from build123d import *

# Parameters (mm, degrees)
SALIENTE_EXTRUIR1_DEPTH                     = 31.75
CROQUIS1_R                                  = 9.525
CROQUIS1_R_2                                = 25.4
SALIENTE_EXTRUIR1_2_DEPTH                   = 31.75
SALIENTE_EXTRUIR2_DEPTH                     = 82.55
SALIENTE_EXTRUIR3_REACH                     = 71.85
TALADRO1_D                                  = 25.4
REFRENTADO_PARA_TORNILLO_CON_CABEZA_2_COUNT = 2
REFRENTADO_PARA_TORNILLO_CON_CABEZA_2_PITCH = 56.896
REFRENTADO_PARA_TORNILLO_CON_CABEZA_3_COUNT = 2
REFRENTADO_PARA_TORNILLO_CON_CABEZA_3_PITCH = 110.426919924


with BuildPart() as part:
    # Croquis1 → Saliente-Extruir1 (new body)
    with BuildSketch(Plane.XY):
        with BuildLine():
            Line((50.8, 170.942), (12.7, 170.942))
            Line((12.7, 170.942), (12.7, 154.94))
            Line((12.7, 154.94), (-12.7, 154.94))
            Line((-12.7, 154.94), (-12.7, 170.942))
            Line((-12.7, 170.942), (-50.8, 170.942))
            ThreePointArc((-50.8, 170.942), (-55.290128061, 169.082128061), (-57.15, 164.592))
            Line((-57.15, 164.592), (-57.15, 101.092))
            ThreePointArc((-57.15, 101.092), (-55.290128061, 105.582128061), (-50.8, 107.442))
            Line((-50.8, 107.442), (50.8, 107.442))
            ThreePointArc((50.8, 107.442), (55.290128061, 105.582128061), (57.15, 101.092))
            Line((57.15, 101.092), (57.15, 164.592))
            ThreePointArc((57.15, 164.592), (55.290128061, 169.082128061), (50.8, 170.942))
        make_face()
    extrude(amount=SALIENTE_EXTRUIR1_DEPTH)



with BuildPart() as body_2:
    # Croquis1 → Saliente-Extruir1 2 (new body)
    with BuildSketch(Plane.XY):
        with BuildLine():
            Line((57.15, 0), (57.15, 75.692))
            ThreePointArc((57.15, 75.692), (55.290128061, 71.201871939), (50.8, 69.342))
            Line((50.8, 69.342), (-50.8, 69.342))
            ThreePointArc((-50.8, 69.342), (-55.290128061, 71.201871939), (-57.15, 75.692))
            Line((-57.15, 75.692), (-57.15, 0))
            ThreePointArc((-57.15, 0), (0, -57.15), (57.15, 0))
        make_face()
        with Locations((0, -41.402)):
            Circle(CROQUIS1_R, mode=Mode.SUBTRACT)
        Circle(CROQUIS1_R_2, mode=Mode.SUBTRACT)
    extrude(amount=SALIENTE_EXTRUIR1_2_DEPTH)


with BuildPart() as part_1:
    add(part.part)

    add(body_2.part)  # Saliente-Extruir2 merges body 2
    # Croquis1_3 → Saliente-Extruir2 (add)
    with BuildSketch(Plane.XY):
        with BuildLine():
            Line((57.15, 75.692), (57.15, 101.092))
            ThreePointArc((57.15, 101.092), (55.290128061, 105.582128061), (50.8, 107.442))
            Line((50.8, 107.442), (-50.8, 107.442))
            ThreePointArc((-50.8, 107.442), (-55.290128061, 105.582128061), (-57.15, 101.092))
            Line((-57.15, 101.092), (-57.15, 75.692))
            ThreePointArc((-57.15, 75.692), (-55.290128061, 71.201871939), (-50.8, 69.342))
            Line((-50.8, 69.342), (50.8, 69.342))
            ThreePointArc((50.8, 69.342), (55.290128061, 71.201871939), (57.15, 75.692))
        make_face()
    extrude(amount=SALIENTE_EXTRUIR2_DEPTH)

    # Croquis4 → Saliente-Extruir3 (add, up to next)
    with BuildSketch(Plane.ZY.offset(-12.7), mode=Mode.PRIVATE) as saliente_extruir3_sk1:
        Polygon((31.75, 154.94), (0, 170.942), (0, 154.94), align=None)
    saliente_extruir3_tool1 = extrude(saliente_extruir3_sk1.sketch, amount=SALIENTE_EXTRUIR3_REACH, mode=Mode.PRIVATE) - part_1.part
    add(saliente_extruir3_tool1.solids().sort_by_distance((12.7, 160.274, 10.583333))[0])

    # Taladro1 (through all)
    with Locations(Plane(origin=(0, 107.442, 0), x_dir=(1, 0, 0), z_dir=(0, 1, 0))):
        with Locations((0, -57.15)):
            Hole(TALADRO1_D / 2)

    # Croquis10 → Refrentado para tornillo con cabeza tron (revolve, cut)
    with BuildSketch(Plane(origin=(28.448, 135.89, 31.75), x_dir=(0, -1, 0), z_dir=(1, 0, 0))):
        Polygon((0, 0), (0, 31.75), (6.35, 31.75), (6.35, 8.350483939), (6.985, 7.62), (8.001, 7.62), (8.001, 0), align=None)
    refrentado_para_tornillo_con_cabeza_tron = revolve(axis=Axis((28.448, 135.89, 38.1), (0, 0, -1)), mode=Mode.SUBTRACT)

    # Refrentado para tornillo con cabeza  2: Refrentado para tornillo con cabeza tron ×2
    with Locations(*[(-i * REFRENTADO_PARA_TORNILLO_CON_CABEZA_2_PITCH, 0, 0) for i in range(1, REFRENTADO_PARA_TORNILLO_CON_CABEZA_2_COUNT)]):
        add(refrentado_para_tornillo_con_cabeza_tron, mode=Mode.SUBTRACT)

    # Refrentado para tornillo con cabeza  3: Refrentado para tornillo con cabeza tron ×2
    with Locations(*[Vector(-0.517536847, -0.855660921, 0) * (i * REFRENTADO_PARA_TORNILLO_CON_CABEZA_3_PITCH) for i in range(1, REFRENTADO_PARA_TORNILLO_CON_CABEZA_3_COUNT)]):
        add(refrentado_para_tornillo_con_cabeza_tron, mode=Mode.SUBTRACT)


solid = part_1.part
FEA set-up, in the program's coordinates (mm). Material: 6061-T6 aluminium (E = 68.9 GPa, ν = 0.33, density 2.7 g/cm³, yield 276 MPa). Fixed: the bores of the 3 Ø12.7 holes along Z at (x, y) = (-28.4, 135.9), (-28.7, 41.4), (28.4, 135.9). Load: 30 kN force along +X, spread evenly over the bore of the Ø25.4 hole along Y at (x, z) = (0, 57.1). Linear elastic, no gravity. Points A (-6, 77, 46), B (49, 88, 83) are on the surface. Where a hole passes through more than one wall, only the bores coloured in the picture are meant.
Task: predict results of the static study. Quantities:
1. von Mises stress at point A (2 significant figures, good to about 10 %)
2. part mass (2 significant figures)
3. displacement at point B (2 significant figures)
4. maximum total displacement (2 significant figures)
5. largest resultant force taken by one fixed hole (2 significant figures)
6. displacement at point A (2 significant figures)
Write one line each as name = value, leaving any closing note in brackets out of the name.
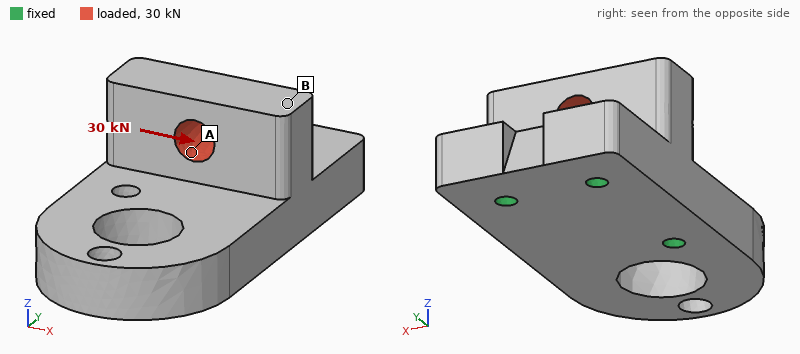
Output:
von Mises stress at point A = 27 MPa
part mass = 2.4 kg
displacement at point B = 0.094 mm
maximum total displacement = 0.10 mm
largest resultant force taken by one fixed hole = 18 kN
displacement at point A = 0.040 mm
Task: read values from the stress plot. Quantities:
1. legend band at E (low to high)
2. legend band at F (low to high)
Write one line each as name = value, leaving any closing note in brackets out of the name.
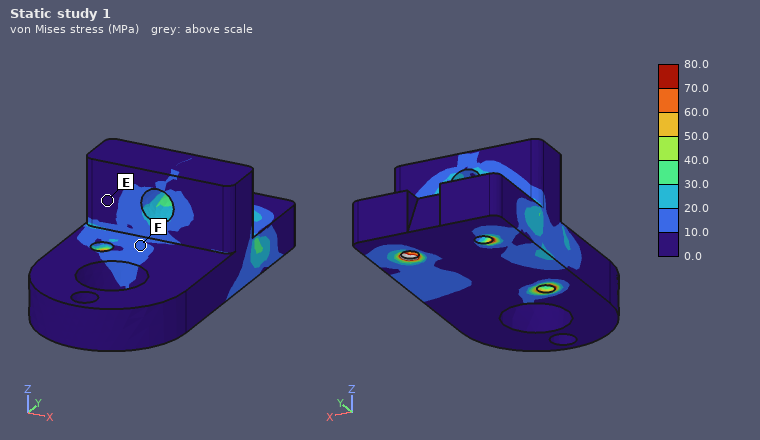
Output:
legend band at E = 0.0 to 10.0 MPa
legend band at F = 10.0 to 20.0 MPa
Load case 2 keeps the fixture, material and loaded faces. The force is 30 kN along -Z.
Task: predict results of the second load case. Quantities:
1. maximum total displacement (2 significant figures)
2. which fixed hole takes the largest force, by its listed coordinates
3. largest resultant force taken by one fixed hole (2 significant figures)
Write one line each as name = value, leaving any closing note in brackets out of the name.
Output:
maximum total displacement = 43 µm
which fixed hole takes the largest force, by its listed coordinates = (-28.7, 41.4)
largest resultant force taken by one fixed hole = 14 kN
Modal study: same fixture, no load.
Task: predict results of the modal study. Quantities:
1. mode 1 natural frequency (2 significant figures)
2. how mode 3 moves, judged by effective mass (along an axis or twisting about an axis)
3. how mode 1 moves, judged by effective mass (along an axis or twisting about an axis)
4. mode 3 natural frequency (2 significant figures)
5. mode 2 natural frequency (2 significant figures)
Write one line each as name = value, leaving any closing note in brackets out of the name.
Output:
mode 1 natural frequency = 1900 Hz
how mode 3 moves, judged by effective mass = along X
how mode 1 moves, judged by effective mass = along Z
mode 3 natural frequency = 3800 Hz
mode 2 natural frequency = 3100 Hz
